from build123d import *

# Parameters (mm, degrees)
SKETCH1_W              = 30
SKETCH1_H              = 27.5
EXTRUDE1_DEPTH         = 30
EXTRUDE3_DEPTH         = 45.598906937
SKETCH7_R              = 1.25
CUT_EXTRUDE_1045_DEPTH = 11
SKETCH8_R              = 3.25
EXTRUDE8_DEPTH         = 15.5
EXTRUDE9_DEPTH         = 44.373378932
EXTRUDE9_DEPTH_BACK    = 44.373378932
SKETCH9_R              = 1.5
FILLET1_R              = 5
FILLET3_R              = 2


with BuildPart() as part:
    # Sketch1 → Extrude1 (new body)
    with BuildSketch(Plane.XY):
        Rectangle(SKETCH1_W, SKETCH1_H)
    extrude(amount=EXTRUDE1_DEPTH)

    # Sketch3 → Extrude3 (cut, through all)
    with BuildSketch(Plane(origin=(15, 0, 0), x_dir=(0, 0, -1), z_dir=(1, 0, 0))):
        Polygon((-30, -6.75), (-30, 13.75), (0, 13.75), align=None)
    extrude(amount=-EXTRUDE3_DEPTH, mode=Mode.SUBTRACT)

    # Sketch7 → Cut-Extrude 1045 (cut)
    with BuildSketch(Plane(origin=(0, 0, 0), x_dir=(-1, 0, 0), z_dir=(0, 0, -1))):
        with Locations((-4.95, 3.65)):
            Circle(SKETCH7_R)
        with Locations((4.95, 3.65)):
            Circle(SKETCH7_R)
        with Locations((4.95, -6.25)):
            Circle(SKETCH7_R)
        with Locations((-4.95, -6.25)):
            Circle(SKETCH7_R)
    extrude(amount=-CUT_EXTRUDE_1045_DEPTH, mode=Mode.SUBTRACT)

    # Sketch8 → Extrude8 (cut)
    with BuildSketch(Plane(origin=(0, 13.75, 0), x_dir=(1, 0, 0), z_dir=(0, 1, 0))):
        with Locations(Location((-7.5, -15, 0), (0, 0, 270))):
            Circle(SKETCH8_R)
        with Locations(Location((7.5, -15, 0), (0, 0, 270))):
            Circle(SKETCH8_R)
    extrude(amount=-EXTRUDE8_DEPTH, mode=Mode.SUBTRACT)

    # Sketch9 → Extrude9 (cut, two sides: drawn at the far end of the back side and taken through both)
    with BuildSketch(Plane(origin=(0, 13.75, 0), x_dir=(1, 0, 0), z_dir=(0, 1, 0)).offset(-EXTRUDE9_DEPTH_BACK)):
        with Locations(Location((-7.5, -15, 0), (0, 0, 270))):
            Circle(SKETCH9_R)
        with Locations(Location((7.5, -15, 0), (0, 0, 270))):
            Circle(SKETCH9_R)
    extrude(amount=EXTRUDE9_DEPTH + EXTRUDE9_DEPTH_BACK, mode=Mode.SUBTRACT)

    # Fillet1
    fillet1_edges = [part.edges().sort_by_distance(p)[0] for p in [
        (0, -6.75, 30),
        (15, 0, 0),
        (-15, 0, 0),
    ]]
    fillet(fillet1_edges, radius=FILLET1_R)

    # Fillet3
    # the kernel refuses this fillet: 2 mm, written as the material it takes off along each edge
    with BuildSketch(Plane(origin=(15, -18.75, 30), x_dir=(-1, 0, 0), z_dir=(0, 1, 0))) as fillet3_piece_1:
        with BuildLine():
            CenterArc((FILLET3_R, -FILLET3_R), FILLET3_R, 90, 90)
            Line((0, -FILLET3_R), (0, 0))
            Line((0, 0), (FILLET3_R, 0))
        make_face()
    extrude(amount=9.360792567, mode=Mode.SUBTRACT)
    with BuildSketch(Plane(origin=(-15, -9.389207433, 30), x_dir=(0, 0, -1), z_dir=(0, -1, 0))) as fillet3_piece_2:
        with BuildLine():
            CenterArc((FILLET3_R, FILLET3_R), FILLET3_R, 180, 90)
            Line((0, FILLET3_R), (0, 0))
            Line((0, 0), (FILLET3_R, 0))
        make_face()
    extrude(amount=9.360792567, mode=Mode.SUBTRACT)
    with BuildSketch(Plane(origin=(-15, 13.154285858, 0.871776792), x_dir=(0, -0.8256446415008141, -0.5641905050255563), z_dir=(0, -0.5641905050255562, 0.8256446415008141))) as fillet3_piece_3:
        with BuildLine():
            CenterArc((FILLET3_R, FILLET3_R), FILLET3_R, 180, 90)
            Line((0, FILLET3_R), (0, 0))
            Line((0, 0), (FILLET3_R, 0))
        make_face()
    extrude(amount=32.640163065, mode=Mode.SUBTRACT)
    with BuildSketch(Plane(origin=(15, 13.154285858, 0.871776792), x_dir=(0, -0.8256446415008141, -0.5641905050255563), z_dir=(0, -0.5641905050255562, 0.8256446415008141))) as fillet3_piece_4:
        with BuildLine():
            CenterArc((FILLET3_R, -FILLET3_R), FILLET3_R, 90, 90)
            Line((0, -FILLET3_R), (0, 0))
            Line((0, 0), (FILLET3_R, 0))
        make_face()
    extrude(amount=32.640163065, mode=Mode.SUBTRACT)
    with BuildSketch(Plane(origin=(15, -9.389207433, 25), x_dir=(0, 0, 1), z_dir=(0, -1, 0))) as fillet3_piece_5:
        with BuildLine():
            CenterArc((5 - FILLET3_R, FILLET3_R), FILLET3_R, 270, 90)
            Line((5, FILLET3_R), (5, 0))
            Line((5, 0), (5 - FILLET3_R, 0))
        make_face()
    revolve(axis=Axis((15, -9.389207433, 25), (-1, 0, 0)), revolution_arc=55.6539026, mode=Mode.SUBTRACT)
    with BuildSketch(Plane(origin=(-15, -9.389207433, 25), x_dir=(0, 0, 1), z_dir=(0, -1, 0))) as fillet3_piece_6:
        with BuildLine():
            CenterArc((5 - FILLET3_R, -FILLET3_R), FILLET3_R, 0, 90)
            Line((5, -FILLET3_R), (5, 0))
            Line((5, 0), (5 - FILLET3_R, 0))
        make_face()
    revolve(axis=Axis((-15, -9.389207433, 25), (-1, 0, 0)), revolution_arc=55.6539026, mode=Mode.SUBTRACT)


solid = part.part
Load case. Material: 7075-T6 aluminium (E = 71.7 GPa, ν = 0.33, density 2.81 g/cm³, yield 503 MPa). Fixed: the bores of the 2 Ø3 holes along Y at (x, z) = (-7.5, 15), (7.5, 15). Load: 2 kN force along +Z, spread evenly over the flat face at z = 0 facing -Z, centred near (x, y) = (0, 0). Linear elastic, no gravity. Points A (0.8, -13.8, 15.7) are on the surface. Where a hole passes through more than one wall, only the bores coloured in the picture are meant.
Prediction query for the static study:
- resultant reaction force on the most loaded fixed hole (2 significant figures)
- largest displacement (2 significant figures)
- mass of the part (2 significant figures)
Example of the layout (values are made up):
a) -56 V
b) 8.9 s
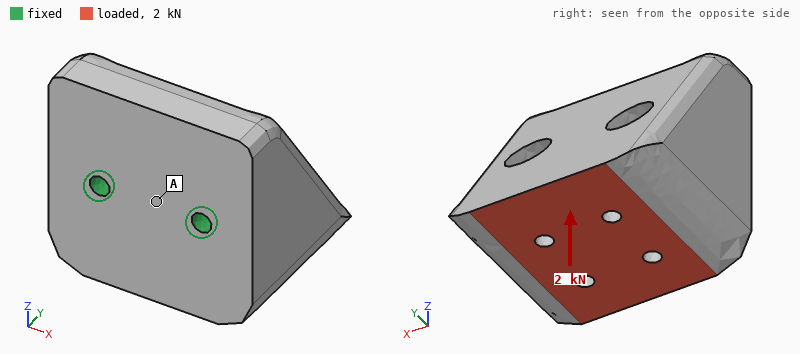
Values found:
a) 1.0 kN
b) 14 µm
c) 40 g
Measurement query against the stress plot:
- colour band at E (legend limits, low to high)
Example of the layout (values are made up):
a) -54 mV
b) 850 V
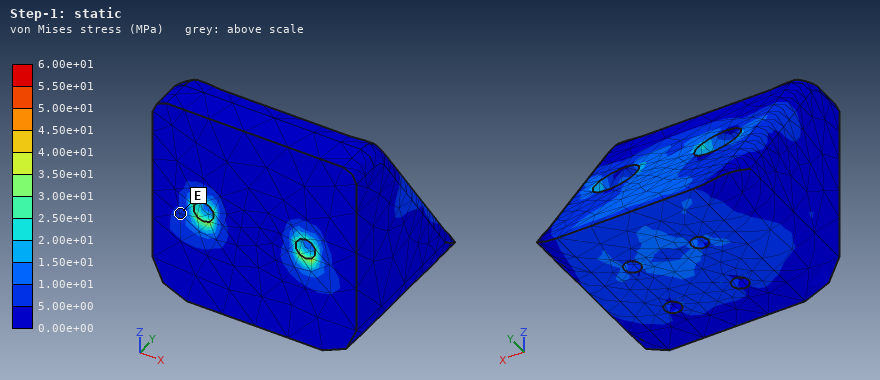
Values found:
a) 5.00e+00 to 1.00e+01 MPa
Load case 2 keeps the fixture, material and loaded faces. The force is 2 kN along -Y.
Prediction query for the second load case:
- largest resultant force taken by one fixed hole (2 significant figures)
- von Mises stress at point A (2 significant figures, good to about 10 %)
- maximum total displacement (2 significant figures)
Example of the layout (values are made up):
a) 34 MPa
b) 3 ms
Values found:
a) 1.0 kN
b) 11 MPa
c) 23 µm
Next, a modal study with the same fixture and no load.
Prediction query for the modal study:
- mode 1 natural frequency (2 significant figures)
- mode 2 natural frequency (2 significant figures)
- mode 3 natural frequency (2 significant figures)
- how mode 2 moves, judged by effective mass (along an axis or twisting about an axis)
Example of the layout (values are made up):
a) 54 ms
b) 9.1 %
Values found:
a) 16 kHz
b) 23 kHz
c) 28 kHz
d) along X
